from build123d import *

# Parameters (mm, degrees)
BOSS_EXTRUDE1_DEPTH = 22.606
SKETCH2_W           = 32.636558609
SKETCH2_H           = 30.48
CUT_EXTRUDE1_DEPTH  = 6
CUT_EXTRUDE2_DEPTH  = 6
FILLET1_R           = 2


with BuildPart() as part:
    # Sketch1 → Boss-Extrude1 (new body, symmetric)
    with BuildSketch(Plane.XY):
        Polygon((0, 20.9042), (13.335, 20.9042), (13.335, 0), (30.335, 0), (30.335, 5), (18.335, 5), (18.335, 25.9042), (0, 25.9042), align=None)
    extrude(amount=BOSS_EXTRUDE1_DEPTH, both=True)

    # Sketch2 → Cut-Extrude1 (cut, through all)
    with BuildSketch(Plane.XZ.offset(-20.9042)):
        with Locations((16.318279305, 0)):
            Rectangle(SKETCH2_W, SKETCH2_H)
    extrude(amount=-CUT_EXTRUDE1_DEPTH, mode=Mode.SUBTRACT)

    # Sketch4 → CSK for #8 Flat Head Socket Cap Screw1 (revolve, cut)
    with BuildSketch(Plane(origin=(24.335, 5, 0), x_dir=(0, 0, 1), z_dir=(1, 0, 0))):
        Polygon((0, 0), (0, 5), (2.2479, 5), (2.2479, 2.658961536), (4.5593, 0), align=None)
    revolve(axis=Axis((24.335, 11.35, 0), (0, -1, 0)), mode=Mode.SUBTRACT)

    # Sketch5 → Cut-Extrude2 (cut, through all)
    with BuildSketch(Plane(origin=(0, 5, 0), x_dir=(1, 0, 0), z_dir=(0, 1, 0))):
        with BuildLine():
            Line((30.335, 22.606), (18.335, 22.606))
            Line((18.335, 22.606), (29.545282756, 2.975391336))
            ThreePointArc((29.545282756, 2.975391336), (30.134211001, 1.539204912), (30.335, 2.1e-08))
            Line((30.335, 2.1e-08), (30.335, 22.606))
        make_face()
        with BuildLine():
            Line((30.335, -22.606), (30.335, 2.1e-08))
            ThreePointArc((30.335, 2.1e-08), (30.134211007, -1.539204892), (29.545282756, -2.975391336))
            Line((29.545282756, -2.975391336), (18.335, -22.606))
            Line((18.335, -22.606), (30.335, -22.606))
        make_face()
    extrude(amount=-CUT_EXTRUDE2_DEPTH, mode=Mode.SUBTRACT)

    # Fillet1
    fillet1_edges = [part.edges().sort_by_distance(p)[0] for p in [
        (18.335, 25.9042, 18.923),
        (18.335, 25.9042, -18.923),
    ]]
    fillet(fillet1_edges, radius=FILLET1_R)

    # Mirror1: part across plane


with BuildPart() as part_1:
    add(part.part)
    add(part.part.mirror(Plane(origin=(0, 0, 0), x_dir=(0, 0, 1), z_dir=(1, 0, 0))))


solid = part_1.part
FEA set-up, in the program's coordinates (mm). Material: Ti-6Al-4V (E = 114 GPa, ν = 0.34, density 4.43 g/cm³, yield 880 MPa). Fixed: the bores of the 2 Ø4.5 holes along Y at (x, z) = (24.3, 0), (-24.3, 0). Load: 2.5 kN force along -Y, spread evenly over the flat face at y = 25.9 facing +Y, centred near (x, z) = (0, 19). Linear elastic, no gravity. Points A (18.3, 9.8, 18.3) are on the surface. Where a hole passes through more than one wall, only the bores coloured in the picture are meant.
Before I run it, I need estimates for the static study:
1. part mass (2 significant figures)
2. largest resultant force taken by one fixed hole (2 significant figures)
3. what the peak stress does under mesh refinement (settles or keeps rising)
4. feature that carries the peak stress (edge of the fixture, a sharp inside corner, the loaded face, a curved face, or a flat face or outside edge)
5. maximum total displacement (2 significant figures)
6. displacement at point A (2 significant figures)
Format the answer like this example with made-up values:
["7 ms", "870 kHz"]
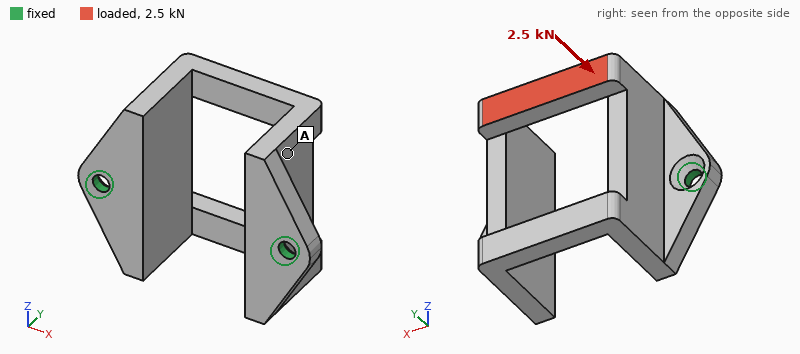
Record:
["65 g", "1.4 kN", "keeps rising", "edge of the fixture", "0.35 mm", "0.19 mm"]
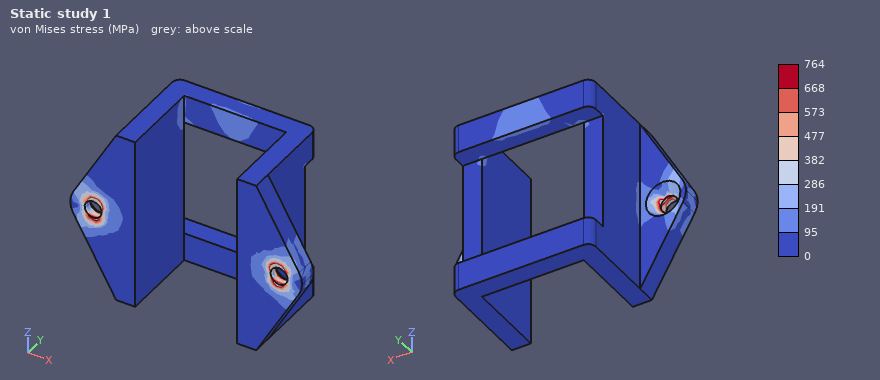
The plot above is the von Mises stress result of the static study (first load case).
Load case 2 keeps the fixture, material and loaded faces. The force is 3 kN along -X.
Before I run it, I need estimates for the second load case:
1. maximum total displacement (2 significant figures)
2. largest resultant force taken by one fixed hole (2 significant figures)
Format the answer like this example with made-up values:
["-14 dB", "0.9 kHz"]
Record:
["0.23 mm", "2.0 kN"]
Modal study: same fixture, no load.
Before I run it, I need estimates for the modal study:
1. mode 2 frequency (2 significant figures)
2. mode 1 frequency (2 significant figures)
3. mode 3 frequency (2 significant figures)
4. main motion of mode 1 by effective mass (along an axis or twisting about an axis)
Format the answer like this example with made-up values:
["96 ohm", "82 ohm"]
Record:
["4600 Hz", "2400 Hz", "4700 Hz", "along Z"]
